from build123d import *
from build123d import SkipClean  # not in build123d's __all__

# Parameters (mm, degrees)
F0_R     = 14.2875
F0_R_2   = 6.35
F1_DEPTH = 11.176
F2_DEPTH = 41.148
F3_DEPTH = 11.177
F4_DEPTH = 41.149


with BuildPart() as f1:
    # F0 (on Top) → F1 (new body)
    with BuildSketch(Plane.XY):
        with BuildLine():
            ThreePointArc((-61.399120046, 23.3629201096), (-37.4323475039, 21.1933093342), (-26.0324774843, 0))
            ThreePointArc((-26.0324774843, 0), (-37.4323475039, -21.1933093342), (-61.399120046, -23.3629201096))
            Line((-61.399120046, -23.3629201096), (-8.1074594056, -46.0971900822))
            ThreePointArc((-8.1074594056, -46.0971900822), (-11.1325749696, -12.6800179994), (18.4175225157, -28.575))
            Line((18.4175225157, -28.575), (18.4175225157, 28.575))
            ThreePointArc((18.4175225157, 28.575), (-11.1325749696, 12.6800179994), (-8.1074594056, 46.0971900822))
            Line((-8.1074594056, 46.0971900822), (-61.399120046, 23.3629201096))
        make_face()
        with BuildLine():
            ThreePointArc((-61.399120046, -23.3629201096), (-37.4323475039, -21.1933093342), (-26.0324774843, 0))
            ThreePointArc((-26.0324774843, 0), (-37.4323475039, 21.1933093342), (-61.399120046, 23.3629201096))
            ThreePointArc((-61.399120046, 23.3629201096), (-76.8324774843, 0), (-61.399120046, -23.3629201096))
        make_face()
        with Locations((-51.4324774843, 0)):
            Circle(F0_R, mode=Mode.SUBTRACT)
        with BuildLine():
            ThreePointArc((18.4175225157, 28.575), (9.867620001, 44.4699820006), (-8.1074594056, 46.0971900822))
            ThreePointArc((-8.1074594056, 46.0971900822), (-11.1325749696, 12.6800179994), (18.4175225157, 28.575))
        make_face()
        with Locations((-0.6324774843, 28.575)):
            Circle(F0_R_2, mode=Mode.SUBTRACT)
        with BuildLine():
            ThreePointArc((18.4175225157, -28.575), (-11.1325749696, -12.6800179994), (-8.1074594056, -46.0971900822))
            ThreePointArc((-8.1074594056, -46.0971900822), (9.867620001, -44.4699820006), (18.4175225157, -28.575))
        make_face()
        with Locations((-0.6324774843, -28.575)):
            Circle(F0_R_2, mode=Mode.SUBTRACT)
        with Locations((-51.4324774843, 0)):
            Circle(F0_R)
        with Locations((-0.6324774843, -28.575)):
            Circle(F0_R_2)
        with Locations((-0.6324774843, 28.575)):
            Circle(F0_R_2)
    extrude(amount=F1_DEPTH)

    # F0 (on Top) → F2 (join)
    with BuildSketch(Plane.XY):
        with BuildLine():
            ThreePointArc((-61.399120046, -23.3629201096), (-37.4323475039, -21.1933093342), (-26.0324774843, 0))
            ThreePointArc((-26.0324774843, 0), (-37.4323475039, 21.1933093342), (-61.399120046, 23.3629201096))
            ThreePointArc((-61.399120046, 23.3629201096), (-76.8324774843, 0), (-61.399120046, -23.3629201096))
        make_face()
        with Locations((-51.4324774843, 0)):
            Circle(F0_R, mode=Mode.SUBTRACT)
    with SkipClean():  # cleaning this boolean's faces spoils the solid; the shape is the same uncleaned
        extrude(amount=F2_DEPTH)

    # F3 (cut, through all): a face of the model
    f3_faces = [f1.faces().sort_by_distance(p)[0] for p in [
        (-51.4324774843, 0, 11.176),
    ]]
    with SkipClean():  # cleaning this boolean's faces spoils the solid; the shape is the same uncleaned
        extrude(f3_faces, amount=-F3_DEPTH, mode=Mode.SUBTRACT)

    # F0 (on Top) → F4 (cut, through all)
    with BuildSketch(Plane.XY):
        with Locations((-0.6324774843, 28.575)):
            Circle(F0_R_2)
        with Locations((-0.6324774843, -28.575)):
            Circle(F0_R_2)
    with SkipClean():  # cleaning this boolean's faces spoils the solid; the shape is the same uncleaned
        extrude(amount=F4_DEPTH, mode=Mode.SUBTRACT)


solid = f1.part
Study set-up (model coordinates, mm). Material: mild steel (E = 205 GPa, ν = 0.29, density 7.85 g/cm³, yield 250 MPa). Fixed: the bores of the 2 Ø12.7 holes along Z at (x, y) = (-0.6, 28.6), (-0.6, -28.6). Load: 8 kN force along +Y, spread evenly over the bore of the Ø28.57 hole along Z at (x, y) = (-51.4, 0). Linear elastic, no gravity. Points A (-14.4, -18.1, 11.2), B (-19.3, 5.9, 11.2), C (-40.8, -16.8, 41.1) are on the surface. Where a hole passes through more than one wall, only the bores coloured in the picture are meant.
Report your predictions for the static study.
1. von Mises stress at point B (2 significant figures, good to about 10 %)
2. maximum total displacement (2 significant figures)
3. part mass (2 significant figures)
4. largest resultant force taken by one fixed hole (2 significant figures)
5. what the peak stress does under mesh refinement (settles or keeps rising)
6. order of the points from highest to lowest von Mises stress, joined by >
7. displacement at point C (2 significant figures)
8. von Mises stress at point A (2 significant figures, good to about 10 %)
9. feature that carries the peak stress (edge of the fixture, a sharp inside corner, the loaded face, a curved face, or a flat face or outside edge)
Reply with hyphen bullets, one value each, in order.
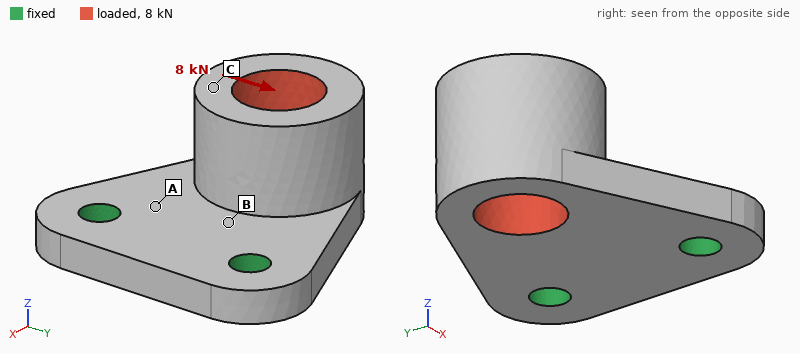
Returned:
- 48 MPa
- 37 µm
- 830 g
- 7.6 kN
- keeps rising
- B > A > C
- 31 µm
- 35 MPa
- edge of the fixture
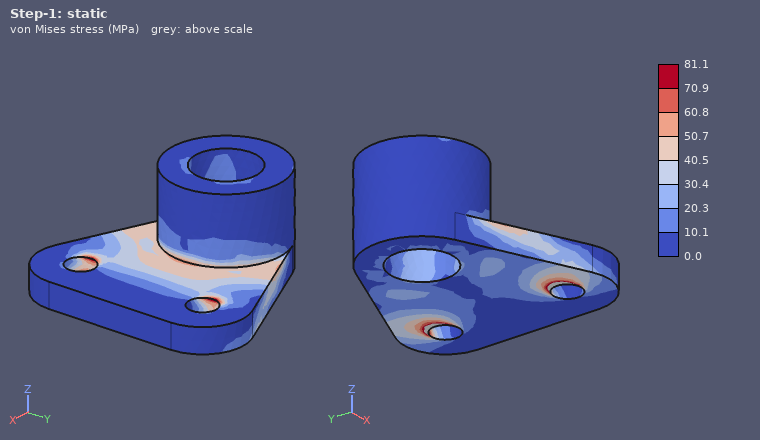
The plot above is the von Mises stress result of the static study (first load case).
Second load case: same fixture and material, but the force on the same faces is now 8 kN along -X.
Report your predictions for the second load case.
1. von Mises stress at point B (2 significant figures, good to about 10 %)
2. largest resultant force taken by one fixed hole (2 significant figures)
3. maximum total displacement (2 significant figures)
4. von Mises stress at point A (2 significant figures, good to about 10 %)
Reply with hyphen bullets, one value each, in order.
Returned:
- 75 MPa
- 4.2 kN
- 0.15 mm
- 72 MPa
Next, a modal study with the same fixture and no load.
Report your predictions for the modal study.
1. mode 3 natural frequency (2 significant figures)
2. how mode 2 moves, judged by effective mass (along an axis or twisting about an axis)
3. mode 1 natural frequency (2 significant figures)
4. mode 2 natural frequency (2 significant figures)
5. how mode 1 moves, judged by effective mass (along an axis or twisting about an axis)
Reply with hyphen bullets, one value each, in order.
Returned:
- 6400 Hz
- along Y
- 1300 Hz
- 3800 Hz
- along Z
